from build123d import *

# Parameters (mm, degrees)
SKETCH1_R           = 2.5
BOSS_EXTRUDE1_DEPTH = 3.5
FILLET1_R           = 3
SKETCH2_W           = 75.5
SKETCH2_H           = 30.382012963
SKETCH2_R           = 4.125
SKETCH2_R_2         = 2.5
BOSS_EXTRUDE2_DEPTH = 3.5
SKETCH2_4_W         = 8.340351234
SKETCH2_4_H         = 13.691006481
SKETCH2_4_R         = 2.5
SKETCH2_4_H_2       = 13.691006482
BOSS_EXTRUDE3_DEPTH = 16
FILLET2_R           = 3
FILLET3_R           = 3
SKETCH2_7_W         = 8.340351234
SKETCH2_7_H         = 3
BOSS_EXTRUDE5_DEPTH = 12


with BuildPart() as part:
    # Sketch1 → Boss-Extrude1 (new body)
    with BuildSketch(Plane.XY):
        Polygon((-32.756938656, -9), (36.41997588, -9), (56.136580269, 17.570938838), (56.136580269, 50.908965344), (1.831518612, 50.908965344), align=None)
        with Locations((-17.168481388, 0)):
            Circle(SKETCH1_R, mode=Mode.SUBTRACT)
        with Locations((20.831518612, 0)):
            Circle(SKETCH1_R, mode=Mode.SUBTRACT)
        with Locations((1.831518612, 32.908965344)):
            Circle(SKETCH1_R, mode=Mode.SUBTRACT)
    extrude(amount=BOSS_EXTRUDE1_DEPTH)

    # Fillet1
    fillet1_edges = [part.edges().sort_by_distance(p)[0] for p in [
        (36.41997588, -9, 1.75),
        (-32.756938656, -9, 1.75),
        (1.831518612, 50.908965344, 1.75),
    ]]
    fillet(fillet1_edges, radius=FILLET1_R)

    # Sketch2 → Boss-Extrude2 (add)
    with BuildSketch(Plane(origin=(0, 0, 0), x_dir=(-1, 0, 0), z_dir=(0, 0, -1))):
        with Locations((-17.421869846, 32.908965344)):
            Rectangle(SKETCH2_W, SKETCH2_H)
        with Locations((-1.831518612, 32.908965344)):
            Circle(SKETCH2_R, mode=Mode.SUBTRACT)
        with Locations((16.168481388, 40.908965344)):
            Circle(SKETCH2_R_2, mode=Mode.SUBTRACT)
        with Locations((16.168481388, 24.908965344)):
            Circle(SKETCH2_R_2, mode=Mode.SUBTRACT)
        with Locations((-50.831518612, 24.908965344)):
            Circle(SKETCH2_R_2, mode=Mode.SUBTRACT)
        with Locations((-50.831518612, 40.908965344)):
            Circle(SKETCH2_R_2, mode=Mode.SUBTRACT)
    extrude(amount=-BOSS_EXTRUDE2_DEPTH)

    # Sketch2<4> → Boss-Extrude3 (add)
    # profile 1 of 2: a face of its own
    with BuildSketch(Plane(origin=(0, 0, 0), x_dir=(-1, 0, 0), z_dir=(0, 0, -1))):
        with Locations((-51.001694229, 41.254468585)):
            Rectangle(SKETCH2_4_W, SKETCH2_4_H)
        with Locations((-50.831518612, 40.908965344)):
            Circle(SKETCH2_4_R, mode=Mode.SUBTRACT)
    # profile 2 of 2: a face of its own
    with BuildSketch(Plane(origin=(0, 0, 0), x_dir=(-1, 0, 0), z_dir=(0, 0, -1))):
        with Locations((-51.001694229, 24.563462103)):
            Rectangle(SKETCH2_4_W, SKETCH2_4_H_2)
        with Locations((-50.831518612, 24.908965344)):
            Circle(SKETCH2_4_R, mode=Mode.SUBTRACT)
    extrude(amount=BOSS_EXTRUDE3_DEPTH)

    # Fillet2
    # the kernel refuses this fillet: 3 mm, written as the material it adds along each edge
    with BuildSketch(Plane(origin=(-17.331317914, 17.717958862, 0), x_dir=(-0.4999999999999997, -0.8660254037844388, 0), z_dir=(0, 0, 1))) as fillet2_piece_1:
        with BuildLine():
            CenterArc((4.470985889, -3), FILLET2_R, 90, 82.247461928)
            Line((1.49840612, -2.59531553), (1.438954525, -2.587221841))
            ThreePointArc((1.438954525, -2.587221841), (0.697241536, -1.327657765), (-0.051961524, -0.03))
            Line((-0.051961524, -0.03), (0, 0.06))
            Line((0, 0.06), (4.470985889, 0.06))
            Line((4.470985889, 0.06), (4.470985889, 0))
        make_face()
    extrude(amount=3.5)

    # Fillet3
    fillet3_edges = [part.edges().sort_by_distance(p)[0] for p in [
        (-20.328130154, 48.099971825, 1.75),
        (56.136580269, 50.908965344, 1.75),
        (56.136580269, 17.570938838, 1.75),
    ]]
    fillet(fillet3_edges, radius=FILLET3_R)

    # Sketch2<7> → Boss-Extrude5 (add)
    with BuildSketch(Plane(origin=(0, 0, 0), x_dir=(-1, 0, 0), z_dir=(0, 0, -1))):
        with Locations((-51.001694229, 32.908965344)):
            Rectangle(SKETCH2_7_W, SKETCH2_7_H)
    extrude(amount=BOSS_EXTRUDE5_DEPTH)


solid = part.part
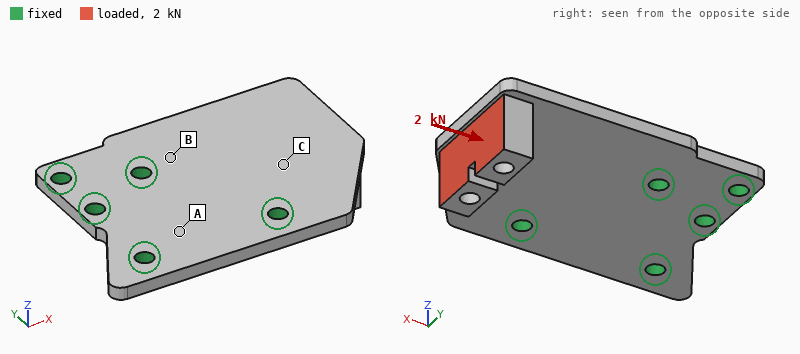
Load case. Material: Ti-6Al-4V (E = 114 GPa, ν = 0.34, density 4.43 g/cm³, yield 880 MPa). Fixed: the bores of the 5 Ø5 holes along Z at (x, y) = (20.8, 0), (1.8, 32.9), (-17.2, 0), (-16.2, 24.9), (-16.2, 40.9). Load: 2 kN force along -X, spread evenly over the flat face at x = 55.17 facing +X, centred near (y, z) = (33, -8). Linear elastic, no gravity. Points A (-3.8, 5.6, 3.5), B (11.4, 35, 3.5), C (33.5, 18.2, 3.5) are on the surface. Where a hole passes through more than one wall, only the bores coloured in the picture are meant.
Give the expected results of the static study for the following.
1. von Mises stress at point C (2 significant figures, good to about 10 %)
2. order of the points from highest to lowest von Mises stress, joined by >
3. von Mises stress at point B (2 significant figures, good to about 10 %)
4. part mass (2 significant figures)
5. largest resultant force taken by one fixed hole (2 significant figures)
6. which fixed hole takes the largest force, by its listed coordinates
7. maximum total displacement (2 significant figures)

150 MPa
C > B > A
71 MPa
81 g
1.1 kN
(1.8, 32.9)
1.0 mm
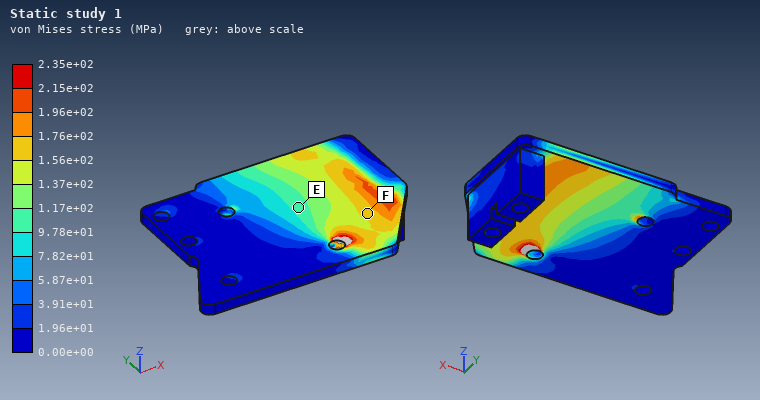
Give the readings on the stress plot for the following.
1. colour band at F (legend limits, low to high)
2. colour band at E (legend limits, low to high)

1.56e+02 to 1.76e+02 MPa
9.78e+01 to 1.17e+02 MPa
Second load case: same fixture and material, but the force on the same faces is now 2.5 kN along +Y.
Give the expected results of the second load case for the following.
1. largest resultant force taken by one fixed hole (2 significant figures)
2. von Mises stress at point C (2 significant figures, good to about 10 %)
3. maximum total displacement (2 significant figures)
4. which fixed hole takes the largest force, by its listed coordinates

3.1 kN
120 MPa
0.83 mm
(20.8, 0)
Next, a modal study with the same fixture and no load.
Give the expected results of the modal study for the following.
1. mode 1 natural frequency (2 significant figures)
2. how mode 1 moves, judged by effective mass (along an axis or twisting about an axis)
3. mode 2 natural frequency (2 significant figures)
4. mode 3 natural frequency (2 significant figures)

930 Hz
along Z
2900 Hz
4500 Hz
